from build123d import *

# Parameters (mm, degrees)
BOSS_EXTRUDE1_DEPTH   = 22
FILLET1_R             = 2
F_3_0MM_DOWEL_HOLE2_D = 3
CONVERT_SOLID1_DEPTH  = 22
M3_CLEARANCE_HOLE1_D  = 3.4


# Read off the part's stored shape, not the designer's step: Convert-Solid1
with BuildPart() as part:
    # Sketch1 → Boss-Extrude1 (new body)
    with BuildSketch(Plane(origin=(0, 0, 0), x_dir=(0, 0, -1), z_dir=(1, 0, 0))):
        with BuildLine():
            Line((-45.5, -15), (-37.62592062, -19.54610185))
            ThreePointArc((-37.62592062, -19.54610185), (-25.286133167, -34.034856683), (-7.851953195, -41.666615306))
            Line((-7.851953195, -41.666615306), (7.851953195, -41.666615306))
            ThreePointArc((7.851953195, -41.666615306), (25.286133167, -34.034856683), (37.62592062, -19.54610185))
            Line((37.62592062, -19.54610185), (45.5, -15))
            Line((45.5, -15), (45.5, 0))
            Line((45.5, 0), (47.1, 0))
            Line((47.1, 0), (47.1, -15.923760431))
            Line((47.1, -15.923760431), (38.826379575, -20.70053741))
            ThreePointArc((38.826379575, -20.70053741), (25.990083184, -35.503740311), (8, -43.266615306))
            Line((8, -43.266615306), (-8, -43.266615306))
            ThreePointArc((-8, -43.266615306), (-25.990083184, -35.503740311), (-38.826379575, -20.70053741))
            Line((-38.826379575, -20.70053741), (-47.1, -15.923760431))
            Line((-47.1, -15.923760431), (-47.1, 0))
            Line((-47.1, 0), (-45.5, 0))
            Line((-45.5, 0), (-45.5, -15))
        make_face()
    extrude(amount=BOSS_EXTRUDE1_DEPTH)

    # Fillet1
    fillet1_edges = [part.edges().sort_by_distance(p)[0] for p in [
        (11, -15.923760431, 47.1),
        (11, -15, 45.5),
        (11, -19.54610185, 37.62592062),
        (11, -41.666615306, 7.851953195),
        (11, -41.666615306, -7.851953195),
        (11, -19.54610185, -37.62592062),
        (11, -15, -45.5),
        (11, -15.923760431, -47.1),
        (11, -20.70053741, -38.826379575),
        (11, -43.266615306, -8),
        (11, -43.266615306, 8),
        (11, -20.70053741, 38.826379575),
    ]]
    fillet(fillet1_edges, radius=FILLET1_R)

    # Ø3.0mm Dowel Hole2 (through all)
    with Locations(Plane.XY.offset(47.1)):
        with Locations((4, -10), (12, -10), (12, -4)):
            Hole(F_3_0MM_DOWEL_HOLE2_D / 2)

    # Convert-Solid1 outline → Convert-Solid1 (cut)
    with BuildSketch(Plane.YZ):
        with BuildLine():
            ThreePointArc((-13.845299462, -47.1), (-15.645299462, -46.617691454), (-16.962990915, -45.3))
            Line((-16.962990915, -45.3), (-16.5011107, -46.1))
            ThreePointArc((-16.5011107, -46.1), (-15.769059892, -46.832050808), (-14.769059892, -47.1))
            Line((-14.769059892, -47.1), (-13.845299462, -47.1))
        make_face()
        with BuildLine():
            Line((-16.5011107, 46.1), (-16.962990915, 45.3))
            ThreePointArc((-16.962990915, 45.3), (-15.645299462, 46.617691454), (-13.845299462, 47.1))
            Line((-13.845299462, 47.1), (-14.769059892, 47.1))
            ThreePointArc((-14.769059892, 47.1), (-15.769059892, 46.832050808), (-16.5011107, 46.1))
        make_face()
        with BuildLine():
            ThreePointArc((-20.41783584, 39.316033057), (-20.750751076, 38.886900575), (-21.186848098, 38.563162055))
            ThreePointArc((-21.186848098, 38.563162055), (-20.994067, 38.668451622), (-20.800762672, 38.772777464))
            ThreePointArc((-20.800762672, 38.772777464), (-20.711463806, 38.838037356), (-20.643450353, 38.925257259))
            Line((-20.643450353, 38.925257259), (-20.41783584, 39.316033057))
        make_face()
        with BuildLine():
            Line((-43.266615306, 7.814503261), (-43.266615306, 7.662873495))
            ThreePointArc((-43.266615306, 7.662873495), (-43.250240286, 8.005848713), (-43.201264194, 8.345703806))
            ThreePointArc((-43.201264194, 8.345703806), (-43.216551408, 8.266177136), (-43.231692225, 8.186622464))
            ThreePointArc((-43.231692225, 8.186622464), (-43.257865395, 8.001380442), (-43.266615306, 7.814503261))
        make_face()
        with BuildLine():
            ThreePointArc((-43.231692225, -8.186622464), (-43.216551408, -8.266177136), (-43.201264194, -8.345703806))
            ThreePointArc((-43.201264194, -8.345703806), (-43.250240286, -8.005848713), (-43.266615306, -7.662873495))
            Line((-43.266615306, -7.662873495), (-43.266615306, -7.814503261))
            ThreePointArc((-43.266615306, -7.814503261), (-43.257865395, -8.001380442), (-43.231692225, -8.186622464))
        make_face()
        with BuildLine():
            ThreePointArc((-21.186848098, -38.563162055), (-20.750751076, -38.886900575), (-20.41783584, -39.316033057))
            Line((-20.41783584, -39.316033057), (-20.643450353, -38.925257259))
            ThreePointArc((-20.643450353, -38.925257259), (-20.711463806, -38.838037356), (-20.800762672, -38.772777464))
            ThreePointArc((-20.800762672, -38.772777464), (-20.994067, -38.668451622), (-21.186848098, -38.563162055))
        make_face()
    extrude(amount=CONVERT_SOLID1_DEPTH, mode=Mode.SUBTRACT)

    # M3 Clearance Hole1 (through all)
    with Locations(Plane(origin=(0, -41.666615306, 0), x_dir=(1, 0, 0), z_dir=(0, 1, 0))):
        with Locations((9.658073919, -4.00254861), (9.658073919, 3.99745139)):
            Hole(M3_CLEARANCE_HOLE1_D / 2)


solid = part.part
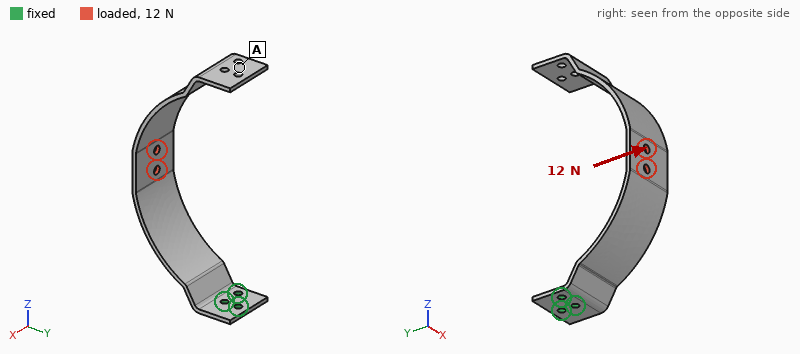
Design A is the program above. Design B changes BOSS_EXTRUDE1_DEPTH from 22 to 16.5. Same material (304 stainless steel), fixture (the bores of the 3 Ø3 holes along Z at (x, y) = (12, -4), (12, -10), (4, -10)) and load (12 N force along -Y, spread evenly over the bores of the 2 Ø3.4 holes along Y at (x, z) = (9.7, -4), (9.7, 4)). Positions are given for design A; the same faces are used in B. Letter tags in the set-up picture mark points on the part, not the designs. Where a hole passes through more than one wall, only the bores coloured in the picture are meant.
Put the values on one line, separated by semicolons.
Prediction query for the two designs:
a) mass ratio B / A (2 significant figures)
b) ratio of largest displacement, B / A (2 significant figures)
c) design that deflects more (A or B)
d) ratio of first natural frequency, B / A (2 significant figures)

0.75; 1.3; B; 1.0
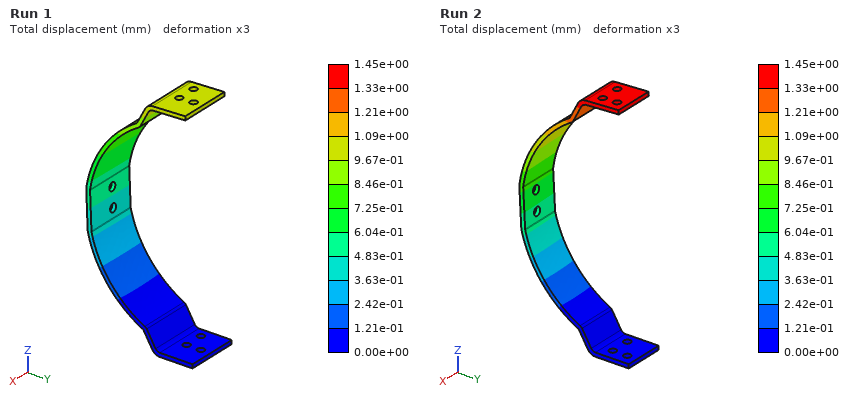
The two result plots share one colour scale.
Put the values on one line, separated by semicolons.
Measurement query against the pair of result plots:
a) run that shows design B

Run 2
